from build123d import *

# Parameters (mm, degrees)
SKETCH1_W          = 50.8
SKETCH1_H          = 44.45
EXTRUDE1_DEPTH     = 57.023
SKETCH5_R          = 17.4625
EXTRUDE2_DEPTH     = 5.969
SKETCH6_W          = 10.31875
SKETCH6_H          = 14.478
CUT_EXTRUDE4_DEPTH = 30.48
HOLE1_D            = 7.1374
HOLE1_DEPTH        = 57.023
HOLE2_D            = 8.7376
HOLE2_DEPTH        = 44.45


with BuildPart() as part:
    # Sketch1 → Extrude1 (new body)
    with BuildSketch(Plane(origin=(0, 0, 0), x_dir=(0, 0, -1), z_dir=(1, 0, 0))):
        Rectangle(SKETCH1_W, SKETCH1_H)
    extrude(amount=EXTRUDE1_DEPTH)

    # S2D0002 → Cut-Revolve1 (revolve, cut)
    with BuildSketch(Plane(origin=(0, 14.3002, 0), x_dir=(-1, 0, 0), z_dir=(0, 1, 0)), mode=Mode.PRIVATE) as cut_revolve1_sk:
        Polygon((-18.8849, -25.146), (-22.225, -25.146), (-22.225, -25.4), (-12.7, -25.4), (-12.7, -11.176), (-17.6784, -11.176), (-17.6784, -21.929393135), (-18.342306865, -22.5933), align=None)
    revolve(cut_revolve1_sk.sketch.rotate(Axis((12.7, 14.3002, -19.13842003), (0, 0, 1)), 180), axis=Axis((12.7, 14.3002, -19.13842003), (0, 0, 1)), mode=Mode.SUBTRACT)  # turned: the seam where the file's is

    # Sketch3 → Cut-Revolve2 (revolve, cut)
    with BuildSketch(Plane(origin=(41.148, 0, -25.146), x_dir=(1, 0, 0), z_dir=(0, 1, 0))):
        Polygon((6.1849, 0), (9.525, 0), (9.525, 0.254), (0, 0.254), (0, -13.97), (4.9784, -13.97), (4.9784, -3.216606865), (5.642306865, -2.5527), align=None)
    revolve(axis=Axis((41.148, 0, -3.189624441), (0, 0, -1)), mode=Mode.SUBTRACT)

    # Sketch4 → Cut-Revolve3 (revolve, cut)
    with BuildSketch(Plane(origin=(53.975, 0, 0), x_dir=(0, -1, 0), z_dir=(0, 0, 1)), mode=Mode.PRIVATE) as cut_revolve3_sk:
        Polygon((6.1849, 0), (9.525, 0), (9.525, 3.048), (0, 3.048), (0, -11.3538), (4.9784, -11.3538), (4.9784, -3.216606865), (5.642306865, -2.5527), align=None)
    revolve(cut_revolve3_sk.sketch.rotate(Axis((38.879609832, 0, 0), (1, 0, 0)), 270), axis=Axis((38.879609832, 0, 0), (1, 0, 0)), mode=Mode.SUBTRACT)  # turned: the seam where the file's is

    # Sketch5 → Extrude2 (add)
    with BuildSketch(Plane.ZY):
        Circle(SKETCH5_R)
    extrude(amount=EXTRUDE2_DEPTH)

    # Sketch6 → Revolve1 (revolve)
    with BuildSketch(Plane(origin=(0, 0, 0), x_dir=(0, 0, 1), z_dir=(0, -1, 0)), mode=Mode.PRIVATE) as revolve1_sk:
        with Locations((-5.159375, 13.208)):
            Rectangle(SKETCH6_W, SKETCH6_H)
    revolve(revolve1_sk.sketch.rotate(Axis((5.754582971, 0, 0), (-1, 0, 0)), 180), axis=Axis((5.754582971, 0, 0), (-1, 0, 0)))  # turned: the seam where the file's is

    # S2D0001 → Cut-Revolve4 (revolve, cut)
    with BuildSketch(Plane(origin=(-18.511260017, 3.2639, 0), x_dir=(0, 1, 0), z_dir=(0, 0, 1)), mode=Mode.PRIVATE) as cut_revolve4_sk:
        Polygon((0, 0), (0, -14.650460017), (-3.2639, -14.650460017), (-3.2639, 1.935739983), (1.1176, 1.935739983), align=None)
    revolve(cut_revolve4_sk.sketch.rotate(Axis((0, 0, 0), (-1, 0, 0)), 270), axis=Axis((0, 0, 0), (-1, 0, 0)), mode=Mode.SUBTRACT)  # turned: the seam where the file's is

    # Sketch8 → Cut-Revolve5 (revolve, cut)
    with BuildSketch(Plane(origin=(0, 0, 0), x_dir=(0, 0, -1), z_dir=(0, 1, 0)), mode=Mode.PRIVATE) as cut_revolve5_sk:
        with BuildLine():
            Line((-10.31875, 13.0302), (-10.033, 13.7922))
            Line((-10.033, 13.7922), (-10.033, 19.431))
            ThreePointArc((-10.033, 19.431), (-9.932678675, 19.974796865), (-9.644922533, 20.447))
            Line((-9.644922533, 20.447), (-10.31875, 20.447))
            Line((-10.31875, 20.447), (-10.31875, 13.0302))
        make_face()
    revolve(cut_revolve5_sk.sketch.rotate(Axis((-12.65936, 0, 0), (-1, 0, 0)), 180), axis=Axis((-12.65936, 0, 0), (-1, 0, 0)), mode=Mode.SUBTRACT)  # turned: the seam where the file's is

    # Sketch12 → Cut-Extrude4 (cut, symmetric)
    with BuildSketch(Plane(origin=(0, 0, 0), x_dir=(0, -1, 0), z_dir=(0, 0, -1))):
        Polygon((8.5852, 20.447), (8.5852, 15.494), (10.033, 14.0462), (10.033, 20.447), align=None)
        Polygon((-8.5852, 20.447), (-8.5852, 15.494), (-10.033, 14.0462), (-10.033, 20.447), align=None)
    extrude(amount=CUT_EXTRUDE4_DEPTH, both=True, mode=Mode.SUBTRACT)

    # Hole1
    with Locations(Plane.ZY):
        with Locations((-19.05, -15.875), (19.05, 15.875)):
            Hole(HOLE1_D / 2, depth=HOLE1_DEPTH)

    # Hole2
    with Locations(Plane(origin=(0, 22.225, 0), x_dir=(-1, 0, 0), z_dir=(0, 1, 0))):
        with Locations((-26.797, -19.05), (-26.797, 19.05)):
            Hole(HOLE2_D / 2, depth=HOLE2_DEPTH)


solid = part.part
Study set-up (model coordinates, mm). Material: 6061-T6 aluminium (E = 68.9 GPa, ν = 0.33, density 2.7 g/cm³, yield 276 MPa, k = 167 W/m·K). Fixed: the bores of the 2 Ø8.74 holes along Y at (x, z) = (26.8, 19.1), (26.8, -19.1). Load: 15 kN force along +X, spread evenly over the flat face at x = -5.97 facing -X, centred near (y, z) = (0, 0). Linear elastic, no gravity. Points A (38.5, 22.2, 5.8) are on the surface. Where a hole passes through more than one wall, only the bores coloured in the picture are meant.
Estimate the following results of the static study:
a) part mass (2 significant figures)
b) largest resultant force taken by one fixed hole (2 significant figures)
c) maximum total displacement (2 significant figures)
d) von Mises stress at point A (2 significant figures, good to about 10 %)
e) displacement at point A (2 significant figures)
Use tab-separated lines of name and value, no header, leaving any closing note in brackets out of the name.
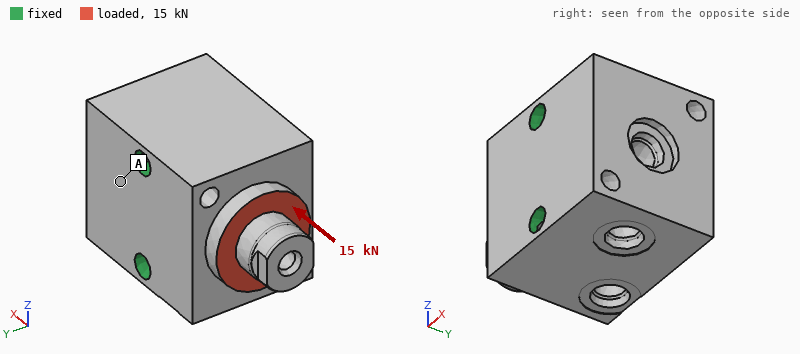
part mass	340 g
largest resultant force taken by one fixed hole	7.7 kN
maximum total displacement	7.1 µm
von Mises stress at point A	3.2 MPa
displacement at point A	1.1 µm
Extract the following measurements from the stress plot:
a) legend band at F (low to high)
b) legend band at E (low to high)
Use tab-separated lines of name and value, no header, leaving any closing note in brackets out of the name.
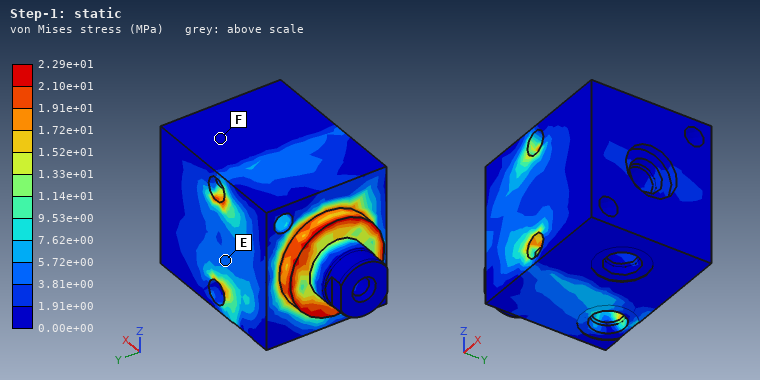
legend band at F	0.00e+00 to 1.91e+00 MPa
legend band at E	3.81e+00 to 5.72e+00 MPa
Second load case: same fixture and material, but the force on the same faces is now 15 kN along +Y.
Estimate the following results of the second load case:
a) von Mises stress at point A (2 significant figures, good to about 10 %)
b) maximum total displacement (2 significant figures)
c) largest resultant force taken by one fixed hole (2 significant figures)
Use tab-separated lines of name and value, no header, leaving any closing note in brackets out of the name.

von Mises stress at point A	9.5 MPa
maximum total displacement	30 µm
largest resultant force taken by one fixed hole	7.7 kN
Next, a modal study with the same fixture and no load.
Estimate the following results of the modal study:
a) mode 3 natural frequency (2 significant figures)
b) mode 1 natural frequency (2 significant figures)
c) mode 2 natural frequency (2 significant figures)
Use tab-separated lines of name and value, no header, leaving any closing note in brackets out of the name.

mode 3 natural frequency	20 kHz
mode 1 natural frequency	16 kHz
mode 2 natural frequency	19 kHz
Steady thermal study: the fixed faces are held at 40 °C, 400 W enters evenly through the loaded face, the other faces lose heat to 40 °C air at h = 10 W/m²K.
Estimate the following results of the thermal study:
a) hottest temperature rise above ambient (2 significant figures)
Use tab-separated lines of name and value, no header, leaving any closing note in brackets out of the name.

hottest temperature rise above ambient	59 K
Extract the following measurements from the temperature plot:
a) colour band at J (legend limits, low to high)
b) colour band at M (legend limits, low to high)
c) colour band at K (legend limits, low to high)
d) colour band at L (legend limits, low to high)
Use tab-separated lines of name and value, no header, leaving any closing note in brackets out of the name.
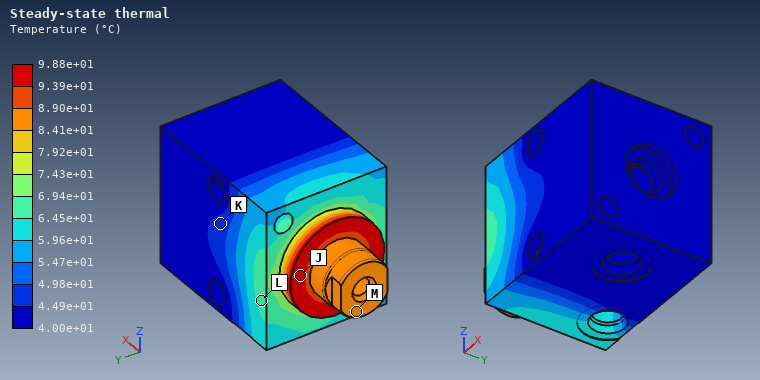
colour band at J	9.39e+01 to 9.88e+01 °C
colour band at M	8.41e+01 to 8.90e+01 °C
colour band at K	4.49e+01 to 4.98e+01 °C
colour band at L	6.45e+01 to 6.94e+01 °C
